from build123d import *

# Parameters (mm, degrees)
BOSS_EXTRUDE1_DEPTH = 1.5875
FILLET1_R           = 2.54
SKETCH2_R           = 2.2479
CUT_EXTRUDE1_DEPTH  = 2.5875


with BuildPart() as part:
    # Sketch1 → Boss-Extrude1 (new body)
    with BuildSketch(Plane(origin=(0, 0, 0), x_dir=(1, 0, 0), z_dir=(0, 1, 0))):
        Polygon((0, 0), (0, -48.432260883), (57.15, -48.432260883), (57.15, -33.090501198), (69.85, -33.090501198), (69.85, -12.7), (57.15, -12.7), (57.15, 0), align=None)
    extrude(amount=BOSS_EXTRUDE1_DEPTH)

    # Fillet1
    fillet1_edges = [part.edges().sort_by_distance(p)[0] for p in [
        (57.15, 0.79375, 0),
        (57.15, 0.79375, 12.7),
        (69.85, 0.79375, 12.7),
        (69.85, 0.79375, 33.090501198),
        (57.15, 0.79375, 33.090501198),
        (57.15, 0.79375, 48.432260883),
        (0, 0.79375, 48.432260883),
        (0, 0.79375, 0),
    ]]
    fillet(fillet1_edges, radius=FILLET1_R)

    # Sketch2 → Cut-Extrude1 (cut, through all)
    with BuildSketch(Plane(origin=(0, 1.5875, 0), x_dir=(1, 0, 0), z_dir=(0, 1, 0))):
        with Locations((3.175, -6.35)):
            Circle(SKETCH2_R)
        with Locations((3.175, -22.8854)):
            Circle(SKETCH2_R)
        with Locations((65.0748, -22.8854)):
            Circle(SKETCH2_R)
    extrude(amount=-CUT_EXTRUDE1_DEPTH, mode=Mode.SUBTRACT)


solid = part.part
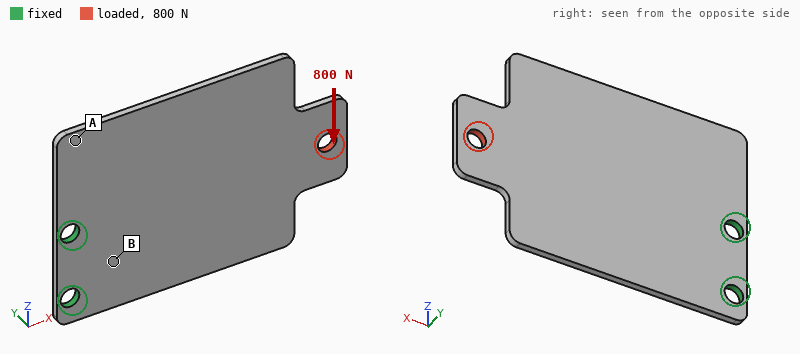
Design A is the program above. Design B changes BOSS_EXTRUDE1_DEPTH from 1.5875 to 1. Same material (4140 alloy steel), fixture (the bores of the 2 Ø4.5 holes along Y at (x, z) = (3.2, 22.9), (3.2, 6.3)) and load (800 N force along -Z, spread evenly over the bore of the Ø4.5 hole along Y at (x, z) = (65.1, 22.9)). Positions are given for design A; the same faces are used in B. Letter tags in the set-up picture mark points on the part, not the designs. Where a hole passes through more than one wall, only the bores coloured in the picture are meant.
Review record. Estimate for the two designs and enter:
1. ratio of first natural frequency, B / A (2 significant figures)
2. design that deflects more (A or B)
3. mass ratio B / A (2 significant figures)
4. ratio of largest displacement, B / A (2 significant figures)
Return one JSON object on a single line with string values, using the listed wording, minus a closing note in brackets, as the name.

{"ratio of first natural frequency, B / A": "0.64", "design that deflects more": "B", "mass ratio B / A": "0.63", "ratio of largest displacement, B / A": "1.6"}
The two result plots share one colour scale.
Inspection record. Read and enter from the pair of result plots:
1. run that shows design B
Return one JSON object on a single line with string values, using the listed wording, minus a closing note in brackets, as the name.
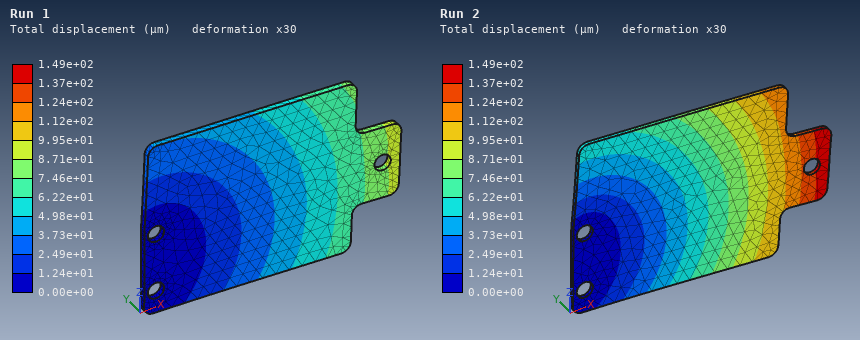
{"run that shows design B": "Run 2"}
